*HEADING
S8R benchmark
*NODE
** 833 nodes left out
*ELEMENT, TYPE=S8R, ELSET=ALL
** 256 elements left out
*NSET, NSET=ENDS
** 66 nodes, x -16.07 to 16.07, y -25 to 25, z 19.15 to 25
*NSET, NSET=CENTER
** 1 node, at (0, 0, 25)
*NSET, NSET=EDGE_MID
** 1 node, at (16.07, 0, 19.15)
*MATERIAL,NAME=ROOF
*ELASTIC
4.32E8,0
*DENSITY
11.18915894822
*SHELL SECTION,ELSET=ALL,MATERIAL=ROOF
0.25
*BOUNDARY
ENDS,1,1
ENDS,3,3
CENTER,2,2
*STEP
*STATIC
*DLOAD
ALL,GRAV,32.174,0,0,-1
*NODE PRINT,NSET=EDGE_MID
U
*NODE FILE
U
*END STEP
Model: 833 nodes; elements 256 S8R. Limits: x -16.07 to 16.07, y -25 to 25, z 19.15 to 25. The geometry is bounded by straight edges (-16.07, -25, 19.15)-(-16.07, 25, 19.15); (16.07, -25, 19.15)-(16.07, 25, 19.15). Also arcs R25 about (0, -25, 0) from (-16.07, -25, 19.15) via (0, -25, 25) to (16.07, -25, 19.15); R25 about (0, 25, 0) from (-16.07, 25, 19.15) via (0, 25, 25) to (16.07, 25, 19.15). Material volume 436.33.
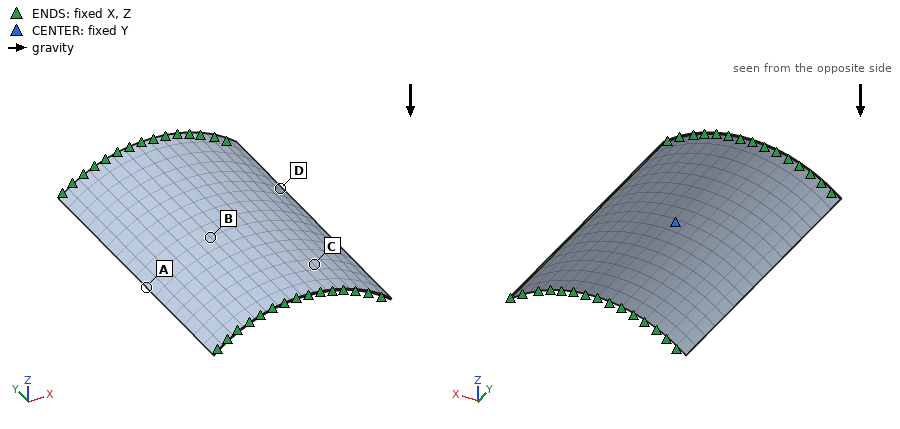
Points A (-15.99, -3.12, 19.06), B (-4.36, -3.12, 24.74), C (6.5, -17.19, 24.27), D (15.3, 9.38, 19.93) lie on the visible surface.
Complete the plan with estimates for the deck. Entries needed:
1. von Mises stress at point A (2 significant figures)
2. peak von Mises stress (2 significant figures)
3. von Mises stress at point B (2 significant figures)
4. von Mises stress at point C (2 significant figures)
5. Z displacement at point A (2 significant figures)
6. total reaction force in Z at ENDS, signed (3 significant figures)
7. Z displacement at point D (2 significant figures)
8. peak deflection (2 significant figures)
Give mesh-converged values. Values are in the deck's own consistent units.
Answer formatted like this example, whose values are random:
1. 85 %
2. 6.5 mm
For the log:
1. 3.6e+05
2. 3.6e+05
3. 1.7e+05
4. 1.5e+05
5. -0.29
6. 1.57e+05
7. -0.24
8. 0.34
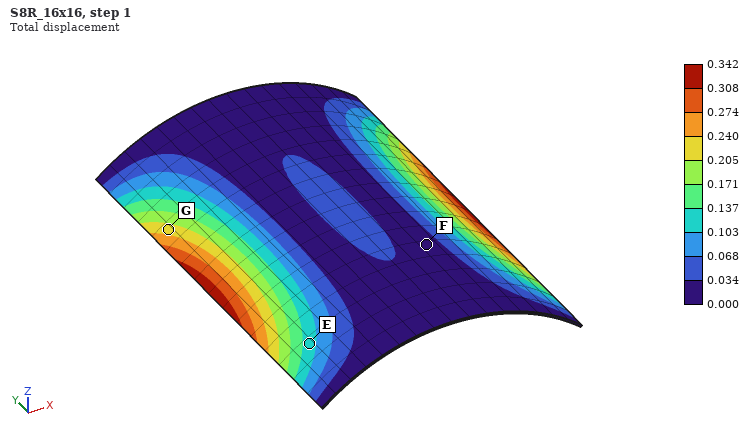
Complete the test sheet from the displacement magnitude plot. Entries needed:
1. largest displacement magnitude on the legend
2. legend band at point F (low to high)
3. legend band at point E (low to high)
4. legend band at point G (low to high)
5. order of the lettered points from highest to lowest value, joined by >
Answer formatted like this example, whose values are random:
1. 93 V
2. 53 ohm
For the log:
1. 0.342
2. 0.000 to 0.034
3. 0.103 to 0.137
4. 0.205 to 0.240
5. G > E > F
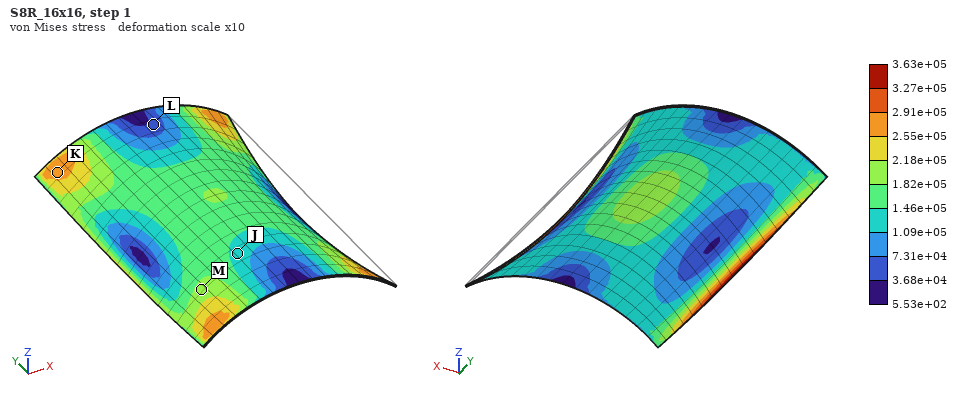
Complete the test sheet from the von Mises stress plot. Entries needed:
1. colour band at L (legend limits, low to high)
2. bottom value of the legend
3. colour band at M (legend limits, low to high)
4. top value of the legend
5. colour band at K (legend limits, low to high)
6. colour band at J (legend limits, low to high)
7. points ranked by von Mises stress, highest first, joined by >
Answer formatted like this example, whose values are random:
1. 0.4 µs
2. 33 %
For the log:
1. 3.68e+04 to 7.31e+04
2. 5.53e+02
3. 1.82e+05 to 2.18e+05
4. 3.63e+05
5. 2.55e+05 to 2.91e+05
6. 1.09e+05 to 1.46e+05
7. K > M > J > L
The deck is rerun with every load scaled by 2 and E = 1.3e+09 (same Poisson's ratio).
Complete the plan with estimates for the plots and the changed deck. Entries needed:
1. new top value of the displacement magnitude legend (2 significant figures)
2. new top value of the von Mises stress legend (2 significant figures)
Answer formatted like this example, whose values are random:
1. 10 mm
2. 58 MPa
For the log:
1. 0.23
2. 7.3e+05
